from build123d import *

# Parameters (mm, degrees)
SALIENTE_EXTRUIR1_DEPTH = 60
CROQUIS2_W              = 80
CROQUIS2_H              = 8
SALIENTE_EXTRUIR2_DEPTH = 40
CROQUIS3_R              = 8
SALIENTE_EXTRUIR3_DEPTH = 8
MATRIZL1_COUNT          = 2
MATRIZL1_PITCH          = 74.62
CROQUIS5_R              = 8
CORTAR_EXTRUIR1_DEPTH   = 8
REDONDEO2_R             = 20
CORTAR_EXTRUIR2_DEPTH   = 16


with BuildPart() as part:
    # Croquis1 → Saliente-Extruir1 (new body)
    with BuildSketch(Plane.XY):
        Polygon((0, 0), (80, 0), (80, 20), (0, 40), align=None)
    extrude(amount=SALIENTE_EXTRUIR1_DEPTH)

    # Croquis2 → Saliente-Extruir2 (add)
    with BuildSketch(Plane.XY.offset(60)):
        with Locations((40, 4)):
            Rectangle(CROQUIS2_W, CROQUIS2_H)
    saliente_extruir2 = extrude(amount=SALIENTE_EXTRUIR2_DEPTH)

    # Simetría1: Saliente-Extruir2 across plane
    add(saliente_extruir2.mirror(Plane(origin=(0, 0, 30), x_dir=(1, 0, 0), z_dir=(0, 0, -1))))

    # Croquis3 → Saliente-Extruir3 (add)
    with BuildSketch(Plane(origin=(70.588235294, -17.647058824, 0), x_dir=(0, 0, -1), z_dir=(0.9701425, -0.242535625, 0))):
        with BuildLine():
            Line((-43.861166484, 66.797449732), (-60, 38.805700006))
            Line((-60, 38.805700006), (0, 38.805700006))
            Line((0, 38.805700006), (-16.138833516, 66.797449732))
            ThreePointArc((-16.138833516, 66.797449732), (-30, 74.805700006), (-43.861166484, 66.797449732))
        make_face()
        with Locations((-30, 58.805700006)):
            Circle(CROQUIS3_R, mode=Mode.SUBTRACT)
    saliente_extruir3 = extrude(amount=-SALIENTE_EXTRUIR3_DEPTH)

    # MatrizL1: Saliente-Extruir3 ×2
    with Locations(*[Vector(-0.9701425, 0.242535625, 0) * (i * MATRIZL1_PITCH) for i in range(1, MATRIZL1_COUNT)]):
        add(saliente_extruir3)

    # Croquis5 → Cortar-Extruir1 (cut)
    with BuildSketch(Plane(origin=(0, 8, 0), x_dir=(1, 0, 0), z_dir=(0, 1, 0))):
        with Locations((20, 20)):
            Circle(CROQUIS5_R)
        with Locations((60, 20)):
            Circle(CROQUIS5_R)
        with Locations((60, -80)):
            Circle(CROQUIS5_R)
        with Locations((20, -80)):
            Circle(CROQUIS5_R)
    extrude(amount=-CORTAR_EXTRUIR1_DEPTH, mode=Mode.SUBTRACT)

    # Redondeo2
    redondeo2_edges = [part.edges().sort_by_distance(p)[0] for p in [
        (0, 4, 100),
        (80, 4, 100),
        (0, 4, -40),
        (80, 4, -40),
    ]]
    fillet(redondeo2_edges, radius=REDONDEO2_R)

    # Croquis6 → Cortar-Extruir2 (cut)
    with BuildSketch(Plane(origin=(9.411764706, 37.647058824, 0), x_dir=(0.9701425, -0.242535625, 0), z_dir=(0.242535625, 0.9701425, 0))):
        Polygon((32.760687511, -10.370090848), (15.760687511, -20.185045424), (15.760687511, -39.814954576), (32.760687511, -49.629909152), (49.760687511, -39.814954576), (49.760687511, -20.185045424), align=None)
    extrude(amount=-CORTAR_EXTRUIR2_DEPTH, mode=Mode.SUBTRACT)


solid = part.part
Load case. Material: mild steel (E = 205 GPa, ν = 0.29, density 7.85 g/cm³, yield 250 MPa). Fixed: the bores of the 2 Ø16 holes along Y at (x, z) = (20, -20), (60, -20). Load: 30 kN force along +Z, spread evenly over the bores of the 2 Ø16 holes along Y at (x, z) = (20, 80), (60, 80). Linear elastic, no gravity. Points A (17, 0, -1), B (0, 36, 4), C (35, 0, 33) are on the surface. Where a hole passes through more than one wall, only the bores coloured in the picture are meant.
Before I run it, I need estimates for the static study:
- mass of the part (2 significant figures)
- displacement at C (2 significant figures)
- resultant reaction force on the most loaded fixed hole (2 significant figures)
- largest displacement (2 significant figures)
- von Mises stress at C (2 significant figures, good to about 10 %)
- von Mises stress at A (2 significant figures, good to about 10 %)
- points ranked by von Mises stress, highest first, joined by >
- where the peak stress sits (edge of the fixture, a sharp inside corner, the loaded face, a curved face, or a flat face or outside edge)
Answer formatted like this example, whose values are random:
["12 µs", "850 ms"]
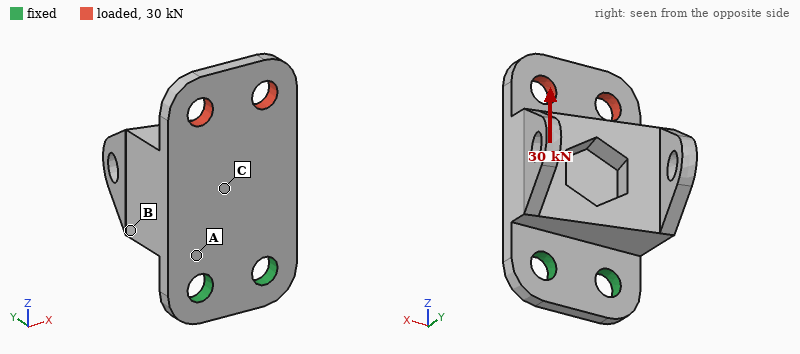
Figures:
["1.5 kg", "15 µm", "15 kN", "62 µm", "41 MPa", "62 MPa", "A > C > B", "the loaded face"]
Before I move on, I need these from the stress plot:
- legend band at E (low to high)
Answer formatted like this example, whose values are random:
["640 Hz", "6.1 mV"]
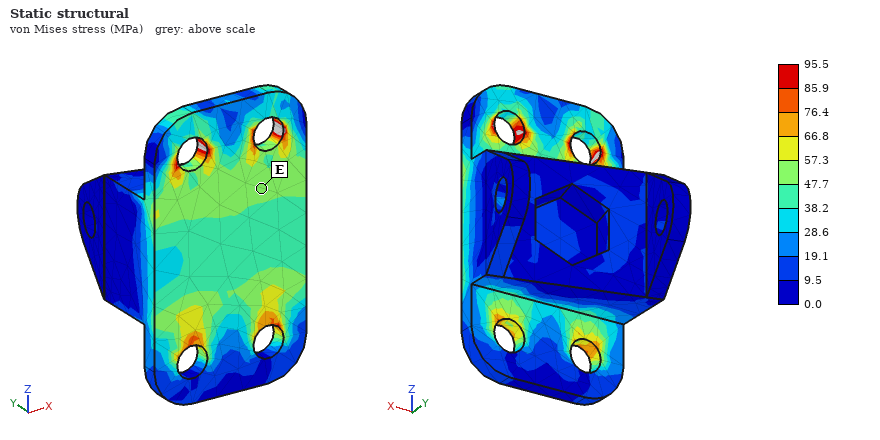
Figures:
["47.7 to 57.3 MPa"]
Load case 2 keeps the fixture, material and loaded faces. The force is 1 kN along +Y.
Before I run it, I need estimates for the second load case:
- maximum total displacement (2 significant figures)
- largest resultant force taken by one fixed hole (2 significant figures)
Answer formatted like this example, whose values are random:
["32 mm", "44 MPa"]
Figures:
["0.26 mm", "510 N"]
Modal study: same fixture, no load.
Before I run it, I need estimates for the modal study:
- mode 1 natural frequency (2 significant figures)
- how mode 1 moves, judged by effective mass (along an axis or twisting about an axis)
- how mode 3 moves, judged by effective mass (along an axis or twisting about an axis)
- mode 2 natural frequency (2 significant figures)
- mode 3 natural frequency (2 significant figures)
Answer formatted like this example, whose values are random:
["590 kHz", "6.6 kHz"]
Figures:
["520 Hz", "along Y", "along X", "2200 Hz", "3000 Hz"]
